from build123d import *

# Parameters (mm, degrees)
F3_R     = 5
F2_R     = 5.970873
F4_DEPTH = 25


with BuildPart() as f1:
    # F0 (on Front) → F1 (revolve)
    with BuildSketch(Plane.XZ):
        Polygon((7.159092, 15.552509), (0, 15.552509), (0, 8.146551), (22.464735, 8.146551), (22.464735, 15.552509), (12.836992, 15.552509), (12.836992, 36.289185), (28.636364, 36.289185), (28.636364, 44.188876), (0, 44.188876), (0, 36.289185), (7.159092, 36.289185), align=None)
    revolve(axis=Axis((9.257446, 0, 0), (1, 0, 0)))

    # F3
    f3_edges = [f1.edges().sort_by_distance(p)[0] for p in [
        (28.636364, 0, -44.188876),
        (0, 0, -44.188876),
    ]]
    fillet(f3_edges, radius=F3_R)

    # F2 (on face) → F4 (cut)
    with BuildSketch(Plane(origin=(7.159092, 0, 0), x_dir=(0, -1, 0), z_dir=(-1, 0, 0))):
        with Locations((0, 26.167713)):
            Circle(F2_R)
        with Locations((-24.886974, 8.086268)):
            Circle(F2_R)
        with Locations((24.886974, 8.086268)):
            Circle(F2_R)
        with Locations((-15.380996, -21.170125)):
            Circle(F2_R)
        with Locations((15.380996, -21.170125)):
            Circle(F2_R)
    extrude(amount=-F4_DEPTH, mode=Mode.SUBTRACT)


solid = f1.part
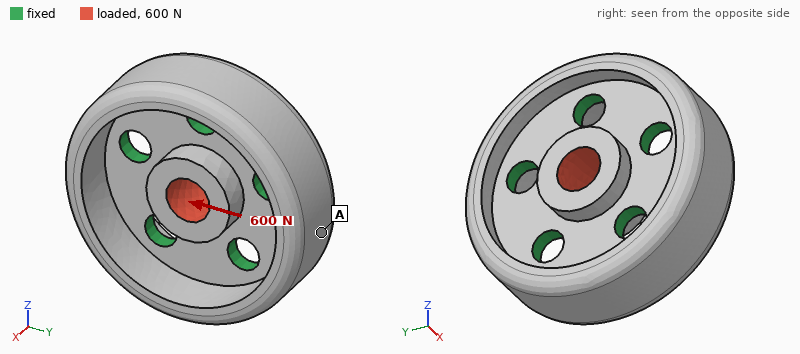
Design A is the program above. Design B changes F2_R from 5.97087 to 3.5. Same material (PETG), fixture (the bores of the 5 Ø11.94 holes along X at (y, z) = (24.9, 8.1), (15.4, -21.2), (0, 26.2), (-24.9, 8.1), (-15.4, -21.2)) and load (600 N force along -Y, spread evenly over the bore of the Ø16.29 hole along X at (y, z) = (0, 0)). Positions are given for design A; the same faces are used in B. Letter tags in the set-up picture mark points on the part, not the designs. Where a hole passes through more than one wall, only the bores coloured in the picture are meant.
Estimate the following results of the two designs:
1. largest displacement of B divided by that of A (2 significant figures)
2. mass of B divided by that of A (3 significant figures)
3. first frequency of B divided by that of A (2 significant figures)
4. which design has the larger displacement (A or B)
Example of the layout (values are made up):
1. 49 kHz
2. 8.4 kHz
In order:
1. 1.2
2. 1.03
3. 0.84
4. B
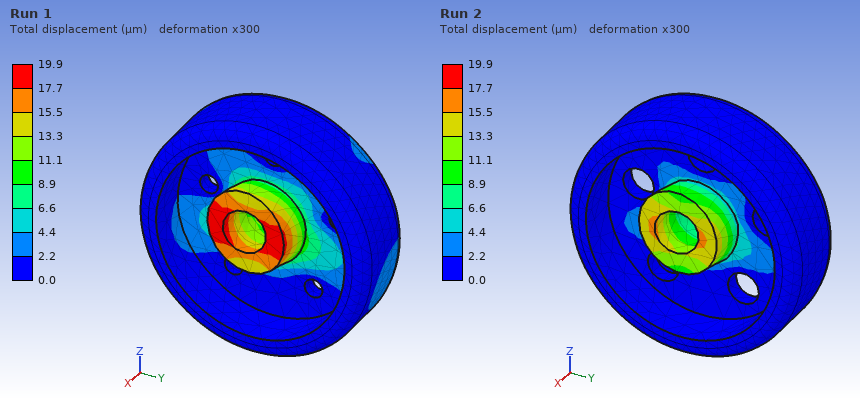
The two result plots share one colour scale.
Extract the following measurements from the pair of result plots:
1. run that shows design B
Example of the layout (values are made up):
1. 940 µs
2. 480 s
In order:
1. Run 1
